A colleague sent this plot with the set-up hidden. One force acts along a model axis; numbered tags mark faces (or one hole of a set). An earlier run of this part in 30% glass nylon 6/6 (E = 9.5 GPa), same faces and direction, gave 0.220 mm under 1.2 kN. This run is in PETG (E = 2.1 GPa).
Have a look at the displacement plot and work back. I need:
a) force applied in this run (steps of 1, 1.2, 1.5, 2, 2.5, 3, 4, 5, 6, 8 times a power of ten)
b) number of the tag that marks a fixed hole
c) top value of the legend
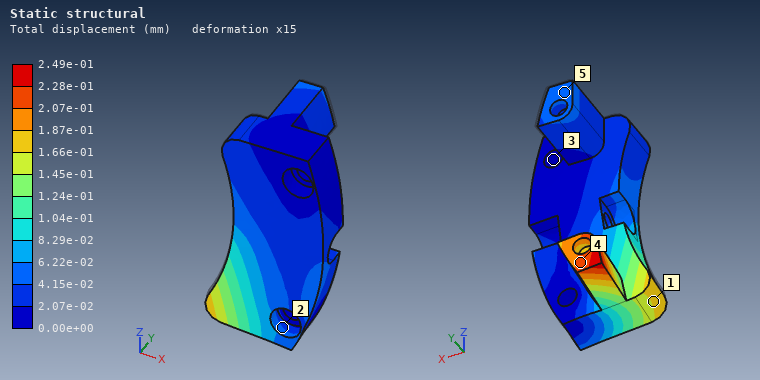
300 N
3
2.49e-01 mm
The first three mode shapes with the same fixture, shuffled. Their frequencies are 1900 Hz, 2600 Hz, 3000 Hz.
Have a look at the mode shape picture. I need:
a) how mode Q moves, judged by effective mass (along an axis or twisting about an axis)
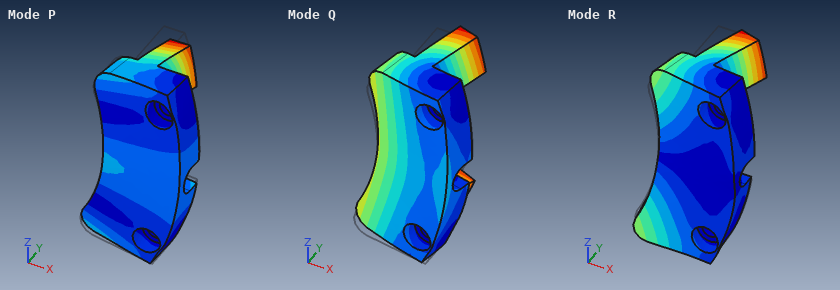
along Y
